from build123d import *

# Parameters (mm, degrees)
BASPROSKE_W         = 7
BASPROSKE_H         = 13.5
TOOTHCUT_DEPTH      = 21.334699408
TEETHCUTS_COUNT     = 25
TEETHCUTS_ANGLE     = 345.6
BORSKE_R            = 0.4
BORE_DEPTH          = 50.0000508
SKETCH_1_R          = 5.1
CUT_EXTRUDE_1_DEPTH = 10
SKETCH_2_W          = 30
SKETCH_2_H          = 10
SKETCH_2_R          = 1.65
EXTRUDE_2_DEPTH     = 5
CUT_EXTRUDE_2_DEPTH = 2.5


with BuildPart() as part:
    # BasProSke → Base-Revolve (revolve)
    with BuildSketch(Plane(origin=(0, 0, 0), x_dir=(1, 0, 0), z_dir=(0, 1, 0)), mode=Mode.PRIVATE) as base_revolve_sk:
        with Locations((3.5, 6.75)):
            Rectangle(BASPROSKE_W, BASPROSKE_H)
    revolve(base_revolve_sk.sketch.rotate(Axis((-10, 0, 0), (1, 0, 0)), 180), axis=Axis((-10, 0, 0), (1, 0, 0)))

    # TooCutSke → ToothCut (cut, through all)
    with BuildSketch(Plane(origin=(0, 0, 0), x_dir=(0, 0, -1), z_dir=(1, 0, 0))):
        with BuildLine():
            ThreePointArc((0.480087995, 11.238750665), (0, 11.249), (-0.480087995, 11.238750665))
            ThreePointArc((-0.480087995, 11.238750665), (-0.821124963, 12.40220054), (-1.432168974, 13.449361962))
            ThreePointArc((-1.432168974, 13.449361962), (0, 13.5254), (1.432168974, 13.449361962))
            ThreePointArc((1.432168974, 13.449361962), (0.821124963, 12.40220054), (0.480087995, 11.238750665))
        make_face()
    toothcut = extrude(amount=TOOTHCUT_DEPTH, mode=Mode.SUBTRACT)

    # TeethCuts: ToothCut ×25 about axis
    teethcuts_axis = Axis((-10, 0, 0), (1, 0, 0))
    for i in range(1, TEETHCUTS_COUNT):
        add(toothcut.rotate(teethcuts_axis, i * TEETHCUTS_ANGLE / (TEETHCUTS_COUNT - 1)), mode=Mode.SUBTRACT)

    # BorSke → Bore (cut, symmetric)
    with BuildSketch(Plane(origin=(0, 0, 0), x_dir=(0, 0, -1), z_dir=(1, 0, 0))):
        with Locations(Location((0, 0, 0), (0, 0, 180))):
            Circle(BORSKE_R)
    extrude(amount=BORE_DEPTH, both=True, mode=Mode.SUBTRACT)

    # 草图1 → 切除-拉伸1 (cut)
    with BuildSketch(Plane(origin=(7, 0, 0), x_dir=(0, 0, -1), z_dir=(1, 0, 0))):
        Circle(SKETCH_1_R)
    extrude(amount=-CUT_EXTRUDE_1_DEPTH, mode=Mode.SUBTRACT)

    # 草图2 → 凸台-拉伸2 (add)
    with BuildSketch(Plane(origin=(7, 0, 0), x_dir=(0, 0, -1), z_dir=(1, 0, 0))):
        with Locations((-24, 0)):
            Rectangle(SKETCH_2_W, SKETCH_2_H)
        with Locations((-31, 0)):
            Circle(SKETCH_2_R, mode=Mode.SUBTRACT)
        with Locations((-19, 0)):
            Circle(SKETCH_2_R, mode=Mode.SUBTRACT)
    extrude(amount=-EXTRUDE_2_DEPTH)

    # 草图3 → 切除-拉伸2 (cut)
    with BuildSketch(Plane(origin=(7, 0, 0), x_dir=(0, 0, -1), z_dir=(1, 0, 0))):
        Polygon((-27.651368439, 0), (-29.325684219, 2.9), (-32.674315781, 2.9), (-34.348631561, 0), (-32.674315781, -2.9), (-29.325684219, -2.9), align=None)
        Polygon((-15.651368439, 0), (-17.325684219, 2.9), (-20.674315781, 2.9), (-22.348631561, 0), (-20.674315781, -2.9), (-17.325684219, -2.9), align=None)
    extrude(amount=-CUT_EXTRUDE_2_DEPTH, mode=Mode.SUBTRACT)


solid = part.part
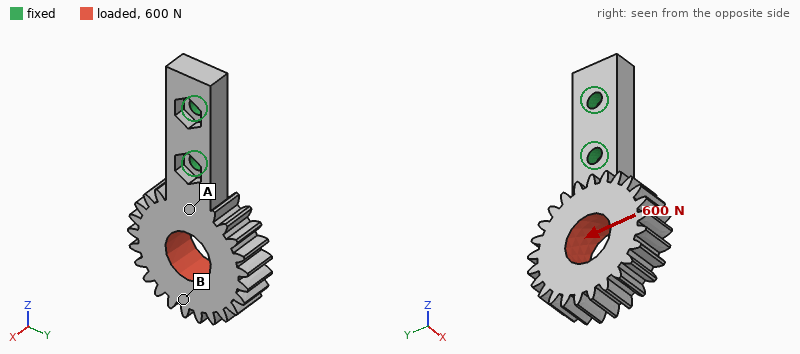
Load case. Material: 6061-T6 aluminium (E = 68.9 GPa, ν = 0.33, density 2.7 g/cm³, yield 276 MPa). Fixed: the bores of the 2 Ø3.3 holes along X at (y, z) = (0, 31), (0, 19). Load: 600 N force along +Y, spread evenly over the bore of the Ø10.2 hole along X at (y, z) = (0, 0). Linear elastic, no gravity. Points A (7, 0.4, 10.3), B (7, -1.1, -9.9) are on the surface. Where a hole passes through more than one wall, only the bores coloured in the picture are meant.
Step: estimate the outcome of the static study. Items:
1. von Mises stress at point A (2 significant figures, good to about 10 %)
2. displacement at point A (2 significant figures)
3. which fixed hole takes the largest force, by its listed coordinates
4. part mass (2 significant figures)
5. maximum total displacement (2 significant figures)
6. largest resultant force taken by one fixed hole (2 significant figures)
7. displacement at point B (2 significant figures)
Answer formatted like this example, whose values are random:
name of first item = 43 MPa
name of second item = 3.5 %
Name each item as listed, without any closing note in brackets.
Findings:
von Mises stress at point A = 45 MPa
displacement at point A = 0.032 mm
which fixed hole takes the largest force, by its listed coordinates = (0, 19)
part mass = 11 g
maximum total displacement = 0.16 mm
largest resultant force taken by one fixed hole = 1.2 kN
displacement at point B = 0.14 mm
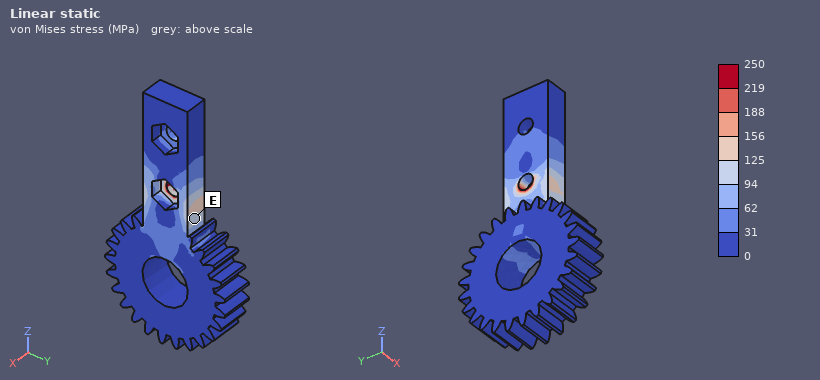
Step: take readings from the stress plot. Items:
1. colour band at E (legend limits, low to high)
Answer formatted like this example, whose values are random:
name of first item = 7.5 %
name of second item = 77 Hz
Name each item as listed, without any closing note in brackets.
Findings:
colour band at E = 94 to 125 MPa
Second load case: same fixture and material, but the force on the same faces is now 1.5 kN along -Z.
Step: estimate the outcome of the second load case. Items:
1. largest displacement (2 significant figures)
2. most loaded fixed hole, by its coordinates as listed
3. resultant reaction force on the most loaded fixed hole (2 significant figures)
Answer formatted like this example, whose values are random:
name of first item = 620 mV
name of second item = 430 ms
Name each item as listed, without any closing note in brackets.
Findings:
largest displacement = 33 µm
most loaded fixed hole, by its coordinates as listed = (0, 19)
resultant reaction force on the most loaded fixed hole = 1.3 kN
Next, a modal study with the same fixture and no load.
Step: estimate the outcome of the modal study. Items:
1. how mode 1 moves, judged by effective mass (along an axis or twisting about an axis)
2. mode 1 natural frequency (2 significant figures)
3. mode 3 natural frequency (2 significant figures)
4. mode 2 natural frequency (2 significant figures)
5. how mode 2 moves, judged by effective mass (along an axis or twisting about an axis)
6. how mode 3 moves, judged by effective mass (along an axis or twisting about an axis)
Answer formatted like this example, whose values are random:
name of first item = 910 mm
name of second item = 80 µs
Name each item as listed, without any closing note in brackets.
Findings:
how mode 1 moves, judged by effective mass = along X
mode 1 natural frequency = 2400 Hz
mode 3 natural frequency = 5900 Hz
mode 2 natural frequency = 4100 Hz
how mode 2 moves, judged by effective mass = along Y
how mode 3 moves, judged by effective mass = twisting about Z
